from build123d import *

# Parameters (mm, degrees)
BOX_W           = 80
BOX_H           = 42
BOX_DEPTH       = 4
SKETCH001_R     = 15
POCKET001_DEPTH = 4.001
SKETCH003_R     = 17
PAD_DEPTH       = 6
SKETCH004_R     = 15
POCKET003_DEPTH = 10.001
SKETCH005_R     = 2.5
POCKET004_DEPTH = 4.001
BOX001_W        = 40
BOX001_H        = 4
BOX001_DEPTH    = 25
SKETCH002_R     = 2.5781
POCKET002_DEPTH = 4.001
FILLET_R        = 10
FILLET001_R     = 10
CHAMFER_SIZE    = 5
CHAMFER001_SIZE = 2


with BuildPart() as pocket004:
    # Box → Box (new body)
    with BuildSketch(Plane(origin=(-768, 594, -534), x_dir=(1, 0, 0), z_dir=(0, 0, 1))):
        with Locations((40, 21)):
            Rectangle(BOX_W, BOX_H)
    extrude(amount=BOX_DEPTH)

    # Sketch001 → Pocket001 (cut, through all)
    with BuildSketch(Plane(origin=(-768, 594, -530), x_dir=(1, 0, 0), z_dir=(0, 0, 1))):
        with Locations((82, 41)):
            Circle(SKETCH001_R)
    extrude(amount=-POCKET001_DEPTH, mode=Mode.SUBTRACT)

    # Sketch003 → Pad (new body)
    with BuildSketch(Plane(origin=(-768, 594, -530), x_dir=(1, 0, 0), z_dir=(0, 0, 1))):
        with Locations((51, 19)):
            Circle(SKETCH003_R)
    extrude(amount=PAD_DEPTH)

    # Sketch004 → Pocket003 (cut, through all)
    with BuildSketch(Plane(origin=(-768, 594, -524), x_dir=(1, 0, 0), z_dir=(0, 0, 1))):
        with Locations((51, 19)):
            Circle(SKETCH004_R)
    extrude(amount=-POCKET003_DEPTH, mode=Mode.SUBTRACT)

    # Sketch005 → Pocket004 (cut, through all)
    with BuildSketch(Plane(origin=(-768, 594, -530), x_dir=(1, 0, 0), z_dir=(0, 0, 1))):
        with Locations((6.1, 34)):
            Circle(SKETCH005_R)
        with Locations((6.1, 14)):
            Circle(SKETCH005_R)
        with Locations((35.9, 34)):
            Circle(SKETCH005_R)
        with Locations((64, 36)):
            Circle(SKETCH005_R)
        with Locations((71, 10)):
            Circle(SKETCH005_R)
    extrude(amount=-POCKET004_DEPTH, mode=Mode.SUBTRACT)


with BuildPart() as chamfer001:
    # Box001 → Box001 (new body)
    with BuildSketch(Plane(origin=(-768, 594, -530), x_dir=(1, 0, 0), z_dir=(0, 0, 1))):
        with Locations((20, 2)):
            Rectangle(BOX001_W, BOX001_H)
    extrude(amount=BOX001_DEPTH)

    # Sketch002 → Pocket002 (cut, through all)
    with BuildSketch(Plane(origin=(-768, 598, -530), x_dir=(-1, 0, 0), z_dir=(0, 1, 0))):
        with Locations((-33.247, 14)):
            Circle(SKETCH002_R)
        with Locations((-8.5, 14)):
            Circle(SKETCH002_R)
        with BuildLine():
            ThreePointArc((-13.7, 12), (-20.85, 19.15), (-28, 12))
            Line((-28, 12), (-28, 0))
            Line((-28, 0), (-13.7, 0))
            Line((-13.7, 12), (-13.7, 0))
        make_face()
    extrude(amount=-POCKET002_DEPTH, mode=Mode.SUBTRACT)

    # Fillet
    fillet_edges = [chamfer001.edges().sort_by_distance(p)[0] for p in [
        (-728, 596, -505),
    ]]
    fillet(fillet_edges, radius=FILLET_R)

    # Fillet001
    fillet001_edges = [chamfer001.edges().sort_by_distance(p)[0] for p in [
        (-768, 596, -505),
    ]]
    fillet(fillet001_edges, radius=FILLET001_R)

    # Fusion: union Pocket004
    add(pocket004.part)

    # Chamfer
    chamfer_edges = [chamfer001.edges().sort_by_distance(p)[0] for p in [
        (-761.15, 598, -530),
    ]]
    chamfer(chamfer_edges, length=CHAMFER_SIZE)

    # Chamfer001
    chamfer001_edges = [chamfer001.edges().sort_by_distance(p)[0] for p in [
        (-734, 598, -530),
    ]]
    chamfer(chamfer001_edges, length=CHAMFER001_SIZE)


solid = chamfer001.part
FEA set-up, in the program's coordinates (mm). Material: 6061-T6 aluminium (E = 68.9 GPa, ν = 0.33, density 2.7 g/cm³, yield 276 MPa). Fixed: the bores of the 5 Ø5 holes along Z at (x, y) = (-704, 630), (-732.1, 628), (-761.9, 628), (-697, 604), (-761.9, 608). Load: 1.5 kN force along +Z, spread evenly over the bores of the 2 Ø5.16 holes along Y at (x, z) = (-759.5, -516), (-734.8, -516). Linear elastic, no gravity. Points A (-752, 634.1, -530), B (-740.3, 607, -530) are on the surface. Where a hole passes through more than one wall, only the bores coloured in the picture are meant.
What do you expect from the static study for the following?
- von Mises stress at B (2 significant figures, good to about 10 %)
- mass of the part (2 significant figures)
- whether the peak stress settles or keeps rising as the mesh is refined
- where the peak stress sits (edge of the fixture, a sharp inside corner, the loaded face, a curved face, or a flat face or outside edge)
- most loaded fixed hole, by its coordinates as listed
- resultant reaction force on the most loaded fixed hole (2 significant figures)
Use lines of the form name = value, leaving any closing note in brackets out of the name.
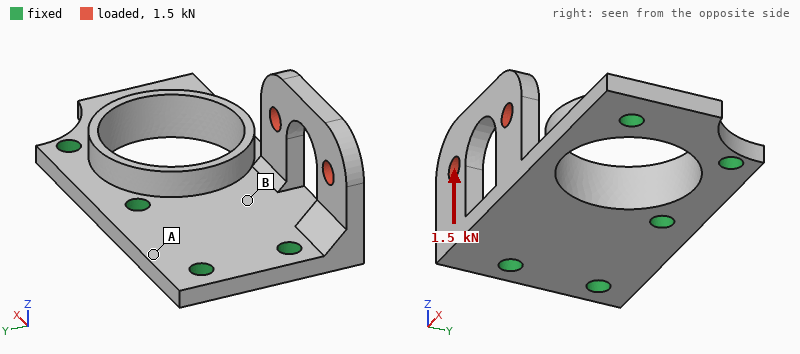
von Mises stress at B = 39 MPa
mass of the part = 37 g
whether the peak stress settles or keeps rising as the mesh is refined = keeps rising
where the peak stress sits = edge of the fixture
most loaded fixed hole, by its coordinates as listed = (-761.9, 608)
resultant reaction force on the most loaded fixed hole = 1.2 kN
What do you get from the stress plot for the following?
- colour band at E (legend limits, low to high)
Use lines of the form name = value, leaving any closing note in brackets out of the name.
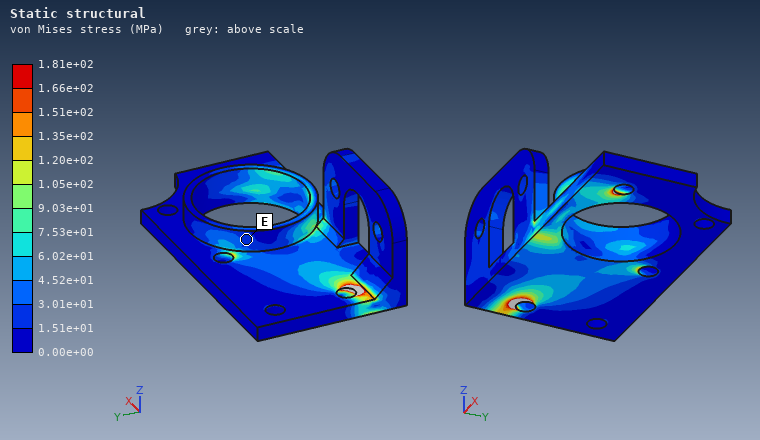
colour band at E = 1.51e+01 to 3.01e+01 MPa
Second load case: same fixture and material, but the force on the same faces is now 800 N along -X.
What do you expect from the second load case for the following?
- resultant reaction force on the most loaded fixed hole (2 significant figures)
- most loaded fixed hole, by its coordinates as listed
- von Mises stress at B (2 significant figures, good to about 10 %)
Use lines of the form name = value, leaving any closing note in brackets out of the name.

resultant reaction force on the most loaded fixed hole = 650 N
most loaded fixed hole, by its coordinates as listed = (-761.9, 608)
von Mises stress at B = 17 MPa
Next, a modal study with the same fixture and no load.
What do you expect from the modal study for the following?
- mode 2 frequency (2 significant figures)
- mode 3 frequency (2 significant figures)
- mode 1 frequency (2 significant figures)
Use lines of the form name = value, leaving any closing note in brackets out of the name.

mode 2 frequency = 5000 Hz
mode 3 frequency = 7200 Hz
mode 1 frequency = 3200 Hz
